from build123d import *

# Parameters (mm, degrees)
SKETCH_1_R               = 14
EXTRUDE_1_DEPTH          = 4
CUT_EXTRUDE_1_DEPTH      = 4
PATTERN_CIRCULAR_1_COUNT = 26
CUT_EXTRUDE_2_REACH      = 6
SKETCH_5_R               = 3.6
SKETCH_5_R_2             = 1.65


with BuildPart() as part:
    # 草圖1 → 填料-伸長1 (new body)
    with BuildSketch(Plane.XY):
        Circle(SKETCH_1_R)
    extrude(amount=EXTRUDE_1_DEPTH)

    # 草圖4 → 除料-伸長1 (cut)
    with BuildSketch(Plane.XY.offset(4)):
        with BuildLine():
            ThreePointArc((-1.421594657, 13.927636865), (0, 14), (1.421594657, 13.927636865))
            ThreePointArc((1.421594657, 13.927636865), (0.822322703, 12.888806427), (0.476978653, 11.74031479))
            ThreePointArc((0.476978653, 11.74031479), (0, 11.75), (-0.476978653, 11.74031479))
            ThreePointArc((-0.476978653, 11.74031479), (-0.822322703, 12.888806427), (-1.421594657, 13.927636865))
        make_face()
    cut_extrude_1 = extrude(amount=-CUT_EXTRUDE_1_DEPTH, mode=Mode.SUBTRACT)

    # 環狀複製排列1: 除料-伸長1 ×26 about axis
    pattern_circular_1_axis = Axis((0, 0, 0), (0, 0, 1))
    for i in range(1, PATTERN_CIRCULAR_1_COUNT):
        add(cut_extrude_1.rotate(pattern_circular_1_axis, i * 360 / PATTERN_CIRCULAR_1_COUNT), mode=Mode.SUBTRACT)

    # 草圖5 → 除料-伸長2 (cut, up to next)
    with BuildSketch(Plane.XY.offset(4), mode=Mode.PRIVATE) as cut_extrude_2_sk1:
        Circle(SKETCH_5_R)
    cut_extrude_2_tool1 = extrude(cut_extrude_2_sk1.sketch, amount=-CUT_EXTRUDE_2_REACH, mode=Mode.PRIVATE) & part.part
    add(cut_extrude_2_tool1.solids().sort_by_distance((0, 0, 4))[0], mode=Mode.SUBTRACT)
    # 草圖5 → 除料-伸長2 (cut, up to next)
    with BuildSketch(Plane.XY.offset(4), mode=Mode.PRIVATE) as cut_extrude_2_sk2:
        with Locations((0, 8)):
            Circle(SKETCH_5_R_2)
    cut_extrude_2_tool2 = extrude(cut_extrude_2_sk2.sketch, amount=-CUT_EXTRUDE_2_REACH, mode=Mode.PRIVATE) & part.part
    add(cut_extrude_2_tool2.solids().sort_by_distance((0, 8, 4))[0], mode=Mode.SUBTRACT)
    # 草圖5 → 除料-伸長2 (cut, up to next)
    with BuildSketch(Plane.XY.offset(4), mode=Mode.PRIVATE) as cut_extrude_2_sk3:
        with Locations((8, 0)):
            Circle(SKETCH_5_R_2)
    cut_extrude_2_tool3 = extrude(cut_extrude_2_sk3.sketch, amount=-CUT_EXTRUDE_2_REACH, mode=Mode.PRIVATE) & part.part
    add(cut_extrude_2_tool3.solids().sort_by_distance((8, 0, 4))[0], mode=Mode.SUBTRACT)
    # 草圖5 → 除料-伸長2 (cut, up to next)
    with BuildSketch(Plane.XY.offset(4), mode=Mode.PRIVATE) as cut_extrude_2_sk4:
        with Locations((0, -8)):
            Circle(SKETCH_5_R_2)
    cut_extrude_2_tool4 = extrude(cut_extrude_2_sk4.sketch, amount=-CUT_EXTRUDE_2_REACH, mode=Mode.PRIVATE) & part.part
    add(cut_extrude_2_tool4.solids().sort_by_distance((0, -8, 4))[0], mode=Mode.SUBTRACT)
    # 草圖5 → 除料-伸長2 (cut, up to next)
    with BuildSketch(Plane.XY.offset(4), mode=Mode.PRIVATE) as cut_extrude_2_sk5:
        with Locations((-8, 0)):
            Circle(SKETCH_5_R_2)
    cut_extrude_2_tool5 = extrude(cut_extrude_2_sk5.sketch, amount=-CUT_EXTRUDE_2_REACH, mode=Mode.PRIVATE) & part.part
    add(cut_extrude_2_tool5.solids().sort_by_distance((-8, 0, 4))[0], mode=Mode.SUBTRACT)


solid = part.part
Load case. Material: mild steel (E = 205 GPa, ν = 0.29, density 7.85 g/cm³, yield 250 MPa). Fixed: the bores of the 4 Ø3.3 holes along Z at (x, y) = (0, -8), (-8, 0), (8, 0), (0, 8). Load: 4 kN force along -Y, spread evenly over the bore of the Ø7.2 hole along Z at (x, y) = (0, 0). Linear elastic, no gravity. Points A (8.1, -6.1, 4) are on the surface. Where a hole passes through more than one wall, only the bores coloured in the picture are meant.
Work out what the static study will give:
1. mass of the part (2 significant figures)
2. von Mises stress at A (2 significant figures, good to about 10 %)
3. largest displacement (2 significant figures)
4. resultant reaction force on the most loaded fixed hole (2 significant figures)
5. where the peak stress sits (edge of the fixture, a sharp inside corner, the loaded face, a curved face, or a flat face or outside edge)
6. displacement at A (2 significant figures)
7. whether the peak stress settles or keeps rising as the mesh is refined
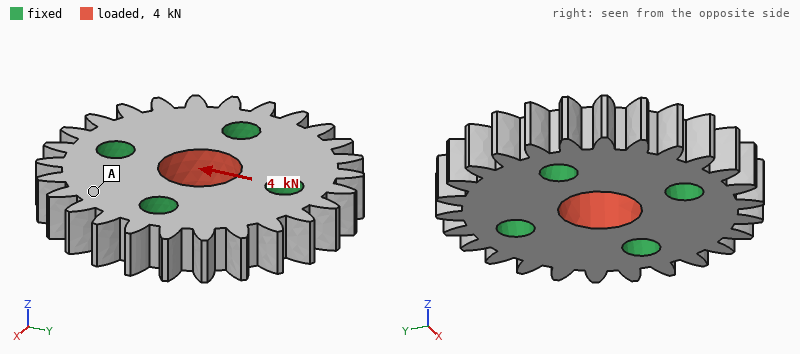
14 g
9.8 MPa
1.3 µm
1.2 kN
edge of the fixture
0.39 µm
keeps rising
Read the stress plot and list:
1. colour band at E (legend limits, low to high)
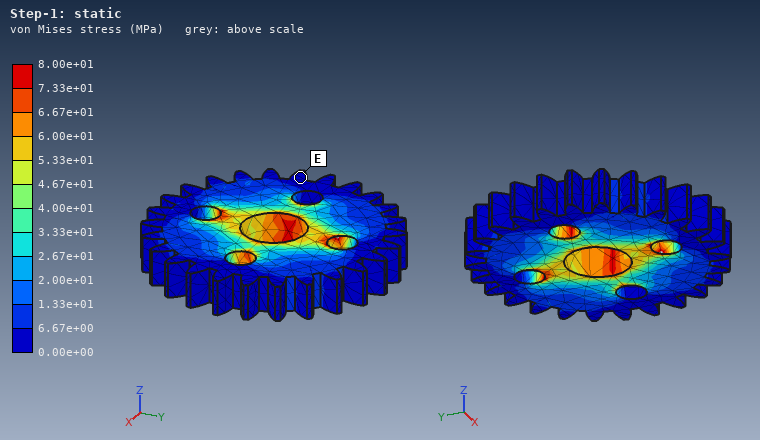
0.00e+00 to 6.67e+00 MPa
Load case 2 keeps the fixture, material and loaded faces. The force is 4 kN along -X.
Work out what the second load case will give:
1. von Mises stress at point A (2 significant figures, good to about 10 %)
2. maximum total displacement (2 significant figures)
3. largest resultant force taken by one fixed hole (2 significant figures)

9.5 MPa
1.3 µm
1.2 kN
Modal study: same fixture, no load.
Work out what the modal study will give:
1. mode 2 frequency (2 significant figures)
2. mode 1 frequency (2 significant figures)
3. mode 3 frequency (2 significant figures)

63 kHz
62 kHz
63 kHz
